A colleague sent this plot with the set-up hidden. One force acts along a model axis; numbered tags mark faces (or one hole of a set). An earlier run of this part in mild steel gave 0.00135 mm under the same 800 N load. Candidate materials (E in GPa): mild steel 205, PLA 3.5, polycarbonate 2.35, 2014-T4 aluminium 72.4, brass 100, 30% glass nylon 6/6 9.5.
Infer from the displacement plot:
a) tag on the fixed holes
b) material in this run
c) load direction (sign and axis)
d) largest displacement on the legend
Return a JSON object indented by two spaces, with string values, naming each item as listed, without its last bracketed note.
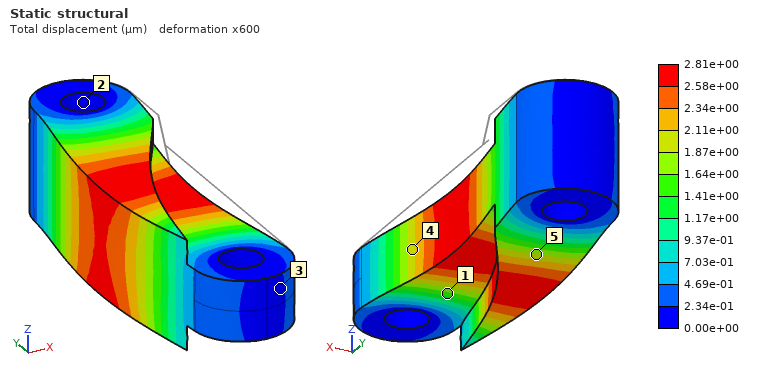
{
  "tag on the fixed holes": "2",
  "material in this run": "brass",
  "load direction": "-X",
  "largest displacement on the legend": "2.81e+00 µm"
}
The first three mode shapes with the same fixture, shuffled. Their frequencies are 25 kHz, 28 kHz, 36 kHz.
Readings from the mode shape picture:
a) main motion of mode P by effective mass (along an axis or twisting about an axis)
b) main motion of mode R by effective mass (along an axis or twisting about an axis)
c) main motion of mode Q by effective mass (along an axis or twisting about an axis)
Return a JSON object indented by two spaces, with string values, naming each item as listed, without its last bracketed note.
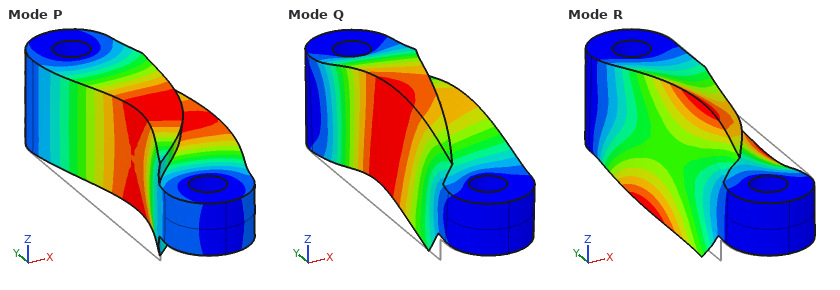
{
  "main motion of mode P by effective mass": "along X",
  "main motion of mode R by effective mass": "twisting about Y",
  "main motion of mode Q by effective mass": "along Z"
}
